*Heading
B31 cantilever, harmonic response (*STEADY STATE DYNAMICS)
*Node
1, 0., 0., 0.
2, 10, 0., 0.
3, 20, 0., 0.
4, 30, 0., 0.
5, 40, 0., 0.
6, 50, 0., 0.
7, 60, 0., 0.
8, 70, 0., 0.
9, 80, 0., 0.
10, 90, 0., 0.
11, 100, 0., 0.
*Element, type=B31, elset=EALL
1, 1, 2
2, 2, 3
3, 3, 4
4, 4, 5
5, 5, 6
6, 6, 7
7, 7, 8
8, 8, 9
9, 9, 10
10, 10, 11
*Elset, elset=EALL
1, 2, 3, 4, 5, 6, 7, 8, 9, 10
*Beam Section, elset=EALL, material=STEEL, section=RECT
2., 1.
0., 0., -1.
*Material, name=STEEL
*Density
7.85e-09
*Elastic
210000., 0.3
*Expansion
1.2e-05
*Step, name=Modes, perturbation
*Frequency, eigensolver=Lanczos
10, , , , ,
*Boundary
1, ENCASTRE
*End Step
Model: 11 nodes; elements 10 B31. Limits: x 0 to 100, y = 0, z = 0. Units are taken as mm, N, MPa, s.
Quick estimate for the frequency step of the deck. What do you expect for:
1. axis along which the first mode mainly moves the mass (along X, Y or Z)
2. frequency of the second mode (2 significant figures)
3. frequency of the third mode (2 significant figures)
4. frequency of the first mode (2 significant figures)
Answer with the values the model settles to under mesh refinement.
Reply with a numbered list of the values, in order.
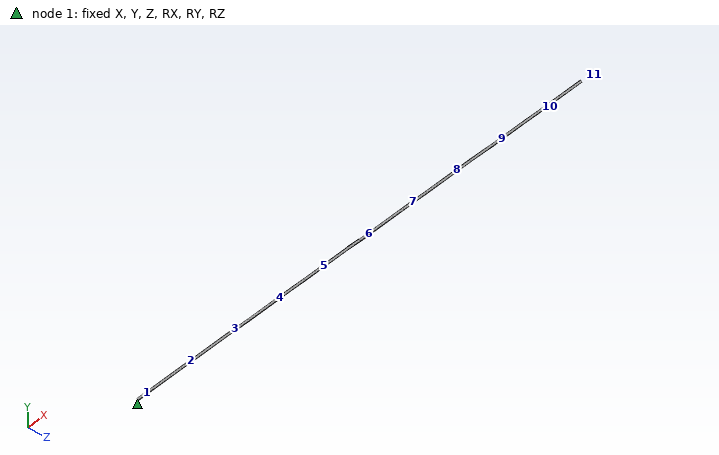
1. along Y
2. 170 Hz
3. 520 Hz
4. 84 Hz
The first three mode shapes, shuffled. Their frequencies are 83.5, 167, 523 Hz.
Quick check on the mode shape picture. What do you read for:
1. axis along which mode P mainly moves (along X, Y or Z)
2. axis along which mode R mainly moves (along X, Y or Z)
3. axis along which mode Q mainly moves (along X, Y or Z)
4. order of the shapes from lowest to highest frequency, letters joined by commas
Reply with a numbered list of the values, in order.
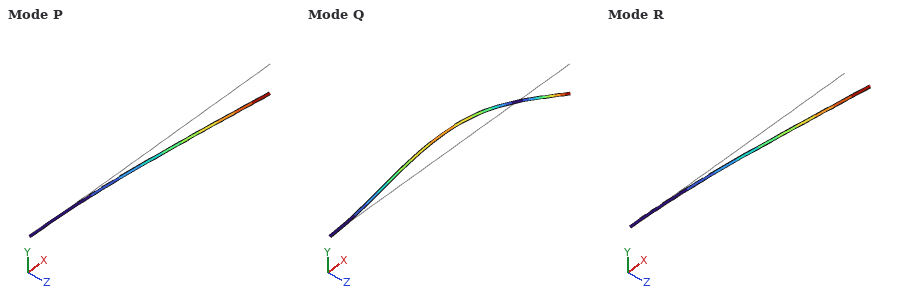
1. along Y
2. along Z
3. along Y
4. P, R, Q
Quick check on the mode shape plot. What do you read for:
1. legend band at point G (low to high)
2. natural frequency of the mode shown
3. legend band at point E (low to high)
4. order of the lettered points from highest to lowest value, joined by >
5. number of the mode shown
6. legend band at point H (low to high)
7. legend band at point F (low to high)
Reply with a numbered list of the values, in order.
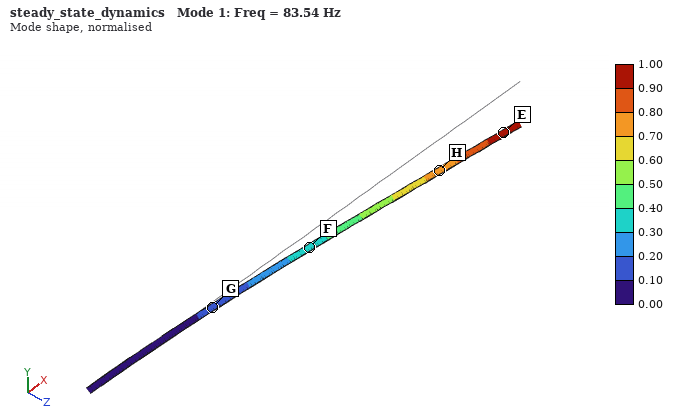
1. 0.10 to 0.20
2. 83.54 Hz
3. 0.90 to 1.00
4. E > H > F > G
5. 1
6. 0.70 to 0.80
7. 0.30 to 0.40
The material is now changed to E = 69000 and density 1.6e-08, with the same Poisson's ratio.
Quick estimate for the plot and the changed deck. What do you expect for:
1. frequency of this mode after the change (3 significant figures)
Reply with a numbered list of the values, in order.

1. 33.5 Hz
